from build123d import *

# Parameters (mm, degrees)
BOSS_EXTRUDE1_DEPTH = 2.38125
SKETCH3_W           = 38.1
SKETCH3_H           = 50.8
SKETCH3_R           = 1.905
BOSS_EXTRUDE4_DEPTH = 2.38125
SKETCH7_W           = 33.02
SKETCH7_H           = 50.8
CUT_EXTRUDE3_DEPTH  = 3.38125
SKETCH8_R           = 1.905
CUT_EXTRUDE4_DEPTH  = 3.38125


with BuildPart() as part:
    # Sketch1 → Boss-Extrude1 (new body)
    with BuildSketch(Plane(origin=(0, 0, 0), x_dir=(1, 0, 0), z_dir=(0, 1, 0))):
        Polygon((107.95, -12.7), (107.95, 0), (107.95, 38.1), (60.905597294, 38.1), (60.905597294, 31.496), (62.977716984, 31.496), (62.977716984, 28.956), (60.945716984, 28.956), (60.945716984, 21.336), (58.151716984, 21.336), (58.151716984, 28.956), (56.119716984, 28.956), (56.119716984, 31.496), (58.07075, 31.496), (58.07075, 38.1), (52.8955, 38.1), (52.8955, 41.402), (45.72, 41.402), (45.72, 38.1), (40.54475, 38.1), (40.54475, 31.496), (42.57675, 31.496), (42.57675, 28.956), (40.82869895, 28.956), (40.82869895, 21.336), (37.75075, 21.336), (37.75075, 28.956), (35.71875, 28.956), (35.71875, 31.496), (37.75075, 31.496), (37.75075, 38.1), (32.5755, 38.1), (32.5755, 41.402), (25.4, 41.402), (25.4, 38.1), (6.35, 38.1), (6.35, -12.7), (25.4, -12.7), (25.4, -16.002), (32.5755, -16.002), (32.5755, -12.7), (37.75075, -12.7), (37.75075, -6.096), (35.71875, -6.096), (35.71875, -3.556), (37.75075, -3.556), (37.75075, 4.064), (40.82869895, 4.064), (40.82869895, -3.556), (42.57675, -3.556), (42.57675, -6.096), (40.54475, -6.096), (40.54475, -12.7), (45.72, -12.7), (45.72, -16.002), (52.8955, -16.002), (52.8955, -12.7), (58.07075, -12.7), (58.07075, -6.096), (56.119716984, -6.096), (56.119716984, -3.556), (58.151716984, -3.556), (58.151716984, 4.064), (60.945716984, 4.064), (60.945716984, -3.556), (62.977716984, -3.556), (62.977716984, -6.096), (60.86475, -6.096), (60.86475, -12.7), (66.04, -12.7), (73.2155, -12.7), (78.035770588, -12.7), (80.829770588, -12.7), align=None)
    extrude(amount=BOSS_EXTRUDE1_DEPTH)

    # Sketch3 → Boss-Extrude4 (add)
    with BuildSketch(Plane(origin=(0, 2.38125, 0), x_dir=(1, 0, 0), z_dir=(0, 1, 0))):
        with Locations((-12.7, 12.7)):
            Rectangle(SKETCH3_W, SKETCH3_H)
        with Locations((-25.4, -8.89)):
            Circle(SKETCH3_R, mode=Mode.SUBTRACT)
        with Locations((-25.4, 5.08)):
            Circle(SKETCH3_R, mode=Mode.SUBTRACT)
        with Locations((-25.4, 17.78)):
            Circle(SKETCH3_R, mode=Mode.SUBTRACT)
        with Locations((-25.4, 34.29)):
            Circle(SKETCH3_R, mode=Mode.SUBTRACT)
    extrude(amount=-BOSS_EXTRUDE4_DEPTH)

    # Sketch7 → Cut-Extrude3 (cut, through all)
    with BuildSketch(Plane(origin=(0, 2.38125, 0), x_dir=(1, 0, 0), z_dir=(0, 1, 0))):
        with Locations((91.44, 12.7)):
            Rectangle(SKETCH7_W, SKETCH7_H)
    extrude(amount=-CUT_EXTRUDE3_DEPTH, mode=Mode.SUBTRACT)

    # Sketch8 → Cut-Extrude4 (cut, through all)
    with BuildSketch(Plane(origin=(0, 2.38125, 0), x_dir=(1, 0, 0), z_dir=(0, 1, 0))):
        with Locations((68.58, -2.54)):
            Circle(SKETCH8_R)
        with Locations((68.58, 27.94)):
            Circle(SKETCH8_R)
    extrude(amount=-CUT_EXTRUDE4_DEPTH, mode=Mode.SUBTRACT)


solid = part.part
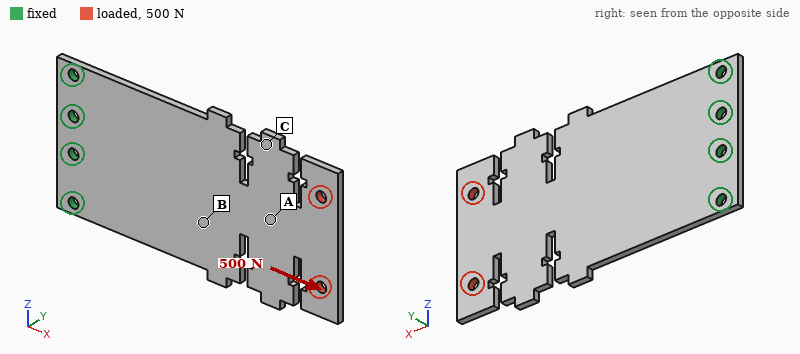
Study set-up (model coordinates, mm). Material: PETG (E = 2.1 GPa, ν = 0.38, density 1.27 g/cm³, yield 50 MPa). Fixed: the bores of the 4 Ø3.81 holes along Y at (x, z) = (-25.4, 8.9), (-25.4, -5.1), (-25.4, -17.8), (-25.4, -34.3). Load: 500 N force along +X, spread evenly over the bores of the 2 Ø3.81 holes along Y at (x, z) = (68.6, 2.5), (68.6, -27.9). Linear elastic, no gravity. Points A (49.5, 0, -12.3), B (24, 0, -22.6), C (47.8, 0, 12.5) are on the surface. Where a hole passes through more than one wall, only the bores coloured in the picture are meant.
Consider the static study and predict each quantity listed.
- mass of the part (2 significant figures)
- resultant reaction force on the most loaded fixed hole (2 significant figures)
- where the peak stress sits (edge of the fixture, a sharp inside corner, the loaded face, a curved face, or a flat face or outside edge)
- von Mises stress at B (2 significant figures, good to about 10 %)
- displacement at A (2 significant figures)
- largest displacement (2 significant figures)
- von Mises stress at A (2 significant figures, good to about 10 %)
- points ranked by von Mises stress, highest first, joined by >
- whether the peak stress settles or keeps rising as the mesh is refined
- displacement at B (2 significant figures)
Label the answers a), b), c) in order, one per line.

a) 16 g
b) 130 N
c) a sharp inside corner
d) 6.3 MPa
e) 0.23 mm
f) 0.68 mm
g) 12 MPa
h) A > B > C
i) keeps rising
j) 0.11 mm
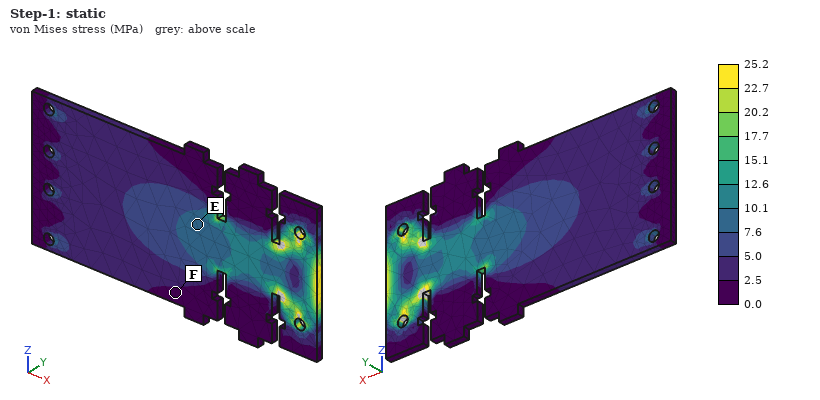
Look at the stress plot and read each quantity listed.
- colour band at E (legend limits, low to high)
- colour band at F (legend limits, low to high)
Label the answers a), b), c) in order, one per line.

a) 7.6 to 10.1 MPa
b) 0.0 to 2.5 MPa
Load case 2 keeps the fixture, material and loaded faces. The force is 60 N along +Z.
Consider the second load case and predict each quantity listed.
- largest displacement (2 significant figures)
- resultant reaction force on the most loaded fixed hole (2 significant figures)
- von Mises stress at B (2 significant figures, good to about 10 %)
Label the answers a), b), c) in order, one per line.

a) 1.0 mm
b) 120 N
c) 3.2 MPa
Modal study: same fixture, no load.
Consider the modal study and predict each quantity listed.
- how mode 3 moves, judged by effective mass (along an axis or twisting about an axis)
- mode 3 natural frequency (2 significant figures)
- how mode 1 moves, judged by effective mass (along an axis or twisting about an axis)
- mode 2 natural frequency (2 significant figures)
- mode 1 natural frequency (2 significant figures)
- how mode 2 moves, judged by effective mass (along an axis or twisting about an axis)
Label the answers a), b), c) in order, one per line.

a) along Y
b) 260 Hz
c) along Y
d) 180 Hz
e) 52 Hz
f) twisting about X
